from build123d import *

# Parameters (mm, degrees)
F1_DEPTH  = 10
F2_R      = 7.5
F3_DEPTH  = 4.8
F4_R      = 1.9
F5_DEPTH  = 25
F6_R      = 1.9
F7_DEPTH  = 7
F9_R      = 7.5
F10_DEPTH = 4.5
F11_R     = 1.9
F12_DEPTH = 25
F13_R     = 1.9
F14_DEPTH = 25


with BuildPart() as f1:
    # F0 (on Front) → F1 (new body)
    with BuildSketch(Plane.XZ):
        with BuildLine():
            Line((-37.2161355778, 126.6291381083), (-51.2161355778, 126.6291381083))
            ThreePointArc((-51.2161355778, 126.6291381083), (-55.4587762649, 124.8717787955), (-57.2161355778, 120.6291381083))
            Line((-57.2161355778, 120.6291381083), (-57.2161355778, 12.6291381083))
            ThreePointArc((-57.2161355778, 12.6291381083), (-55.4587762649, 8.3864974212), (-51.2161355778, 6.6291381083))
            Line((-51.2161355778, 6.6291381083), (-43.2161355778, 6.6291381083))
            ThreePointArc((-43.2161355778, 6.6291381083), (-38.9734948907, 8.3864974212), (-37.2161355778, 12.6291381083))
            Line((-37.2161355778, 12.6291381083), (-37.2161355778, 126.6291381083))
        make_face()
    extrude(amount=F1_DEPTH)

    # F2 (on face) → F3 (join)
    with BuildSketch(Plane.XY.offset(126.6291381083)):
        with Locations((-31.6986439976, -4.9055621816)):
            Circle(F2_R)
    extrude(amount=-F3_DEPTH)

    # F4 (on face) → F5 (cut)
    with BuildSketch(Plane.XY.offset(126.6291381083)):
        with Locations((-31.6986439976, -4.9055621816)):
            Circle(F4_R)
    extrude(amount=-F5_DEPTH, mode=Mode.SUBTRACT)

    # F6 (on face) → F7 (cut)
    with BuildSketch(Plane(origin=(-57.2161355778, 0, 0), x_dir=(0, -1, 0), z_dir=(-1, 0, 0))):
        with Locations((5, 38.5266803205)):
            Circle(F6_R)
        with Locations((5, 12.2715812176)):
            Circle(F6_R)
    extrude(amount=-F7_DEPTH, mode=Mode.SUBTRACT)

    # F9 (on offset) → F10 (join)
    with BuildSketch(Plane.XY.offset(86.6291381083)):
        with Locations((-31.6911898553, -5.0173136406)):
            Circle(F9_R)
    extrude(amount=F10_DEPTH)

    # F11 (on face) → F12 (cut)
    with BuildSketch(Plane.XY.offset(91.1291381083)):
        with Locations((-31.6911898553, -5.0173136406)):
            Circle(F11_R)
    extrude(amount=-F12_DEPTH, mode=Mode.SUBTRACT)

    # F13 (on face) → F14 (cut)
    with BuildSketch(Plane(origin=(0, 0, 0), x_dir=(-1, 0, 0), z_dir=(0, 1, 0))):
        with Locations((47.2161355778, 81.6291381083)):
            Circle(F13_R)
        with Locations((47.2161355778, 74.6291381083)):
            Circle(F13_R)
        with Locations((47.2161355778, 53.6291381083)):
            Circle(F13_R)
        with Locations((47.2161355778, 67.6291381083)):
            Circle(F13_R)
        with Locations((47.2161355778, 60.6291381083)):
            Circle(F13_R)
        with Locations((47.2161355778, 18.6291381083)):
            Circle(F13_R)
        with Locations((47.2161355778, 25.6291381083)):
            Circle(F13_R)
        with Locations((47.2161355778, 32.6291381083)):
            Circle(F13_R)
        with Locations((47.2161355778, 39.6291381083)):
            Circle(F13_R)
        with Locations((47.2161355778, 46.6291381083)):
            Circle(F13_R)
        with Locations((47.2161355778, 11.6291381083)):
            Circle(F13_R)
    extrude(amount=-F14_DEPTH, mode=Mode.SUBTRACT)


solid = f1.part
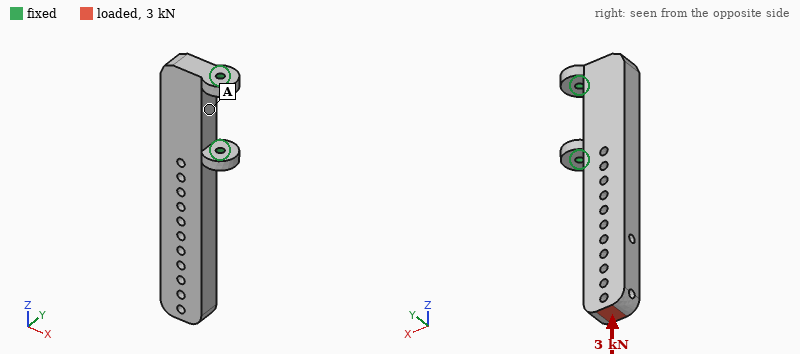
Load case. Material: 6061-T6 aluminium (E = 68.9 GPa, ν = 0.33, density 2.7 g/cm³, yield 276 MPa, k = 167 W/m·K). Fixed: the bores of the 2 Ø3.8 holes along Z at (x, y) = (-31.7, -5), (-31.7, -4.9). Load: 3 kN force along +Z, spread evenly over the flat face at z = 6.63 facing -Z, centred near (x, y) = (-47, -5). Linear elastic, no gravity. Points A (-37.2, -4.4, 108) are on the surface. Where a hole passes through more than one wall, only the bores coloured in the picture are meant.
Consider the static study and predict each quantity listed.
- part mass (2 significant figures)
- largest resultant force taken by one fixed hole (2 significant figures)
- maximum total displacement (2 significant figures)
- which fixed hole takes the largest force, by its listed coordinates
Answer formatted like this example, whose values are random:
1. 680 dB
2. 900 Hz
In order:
1. 64 g
2. 1.9 kN
3. 70 µm
4. (-31.7, -5)
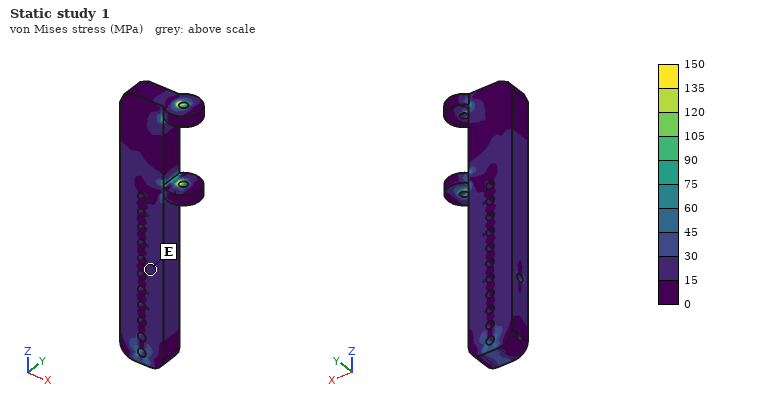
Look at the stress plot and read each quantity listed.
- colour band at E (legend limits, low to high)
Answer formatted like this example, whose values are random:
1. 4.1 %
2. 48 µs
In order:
1. 15 to 30 MPa
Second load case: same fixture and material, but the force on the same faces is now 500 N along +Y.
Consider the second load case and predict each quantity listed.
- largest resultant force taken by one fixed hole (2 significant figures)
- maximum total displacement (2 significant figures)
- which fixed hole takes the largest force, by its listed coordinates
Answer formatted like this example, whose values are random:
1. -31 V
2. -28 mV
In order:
1. 1.5 kN
2. 1.4 mm
3. (-31.7, -5)
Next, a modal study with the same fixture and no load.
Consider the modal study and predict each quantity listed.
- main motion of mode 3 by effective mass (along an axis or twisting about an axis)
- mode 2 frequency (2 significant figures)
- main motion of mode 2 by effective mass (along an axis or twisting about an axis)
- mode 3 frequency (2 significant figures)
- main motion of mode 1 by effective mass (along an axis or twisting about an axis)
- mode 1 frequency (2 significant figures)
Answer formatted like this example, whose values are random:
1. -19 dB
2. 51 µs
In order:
1. along Y
2. 1900 Hz
3. along X
4. 3500 Hz
5. along Y
6. 910 Hz
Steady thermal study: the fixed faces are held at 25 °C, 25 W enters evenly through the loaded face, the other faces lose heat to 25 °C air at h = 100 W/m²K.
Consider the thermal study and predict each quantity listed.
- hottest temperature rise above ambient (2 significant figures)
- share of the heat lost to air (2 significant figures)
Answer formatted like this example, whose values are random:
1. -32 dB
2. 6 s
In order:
1. 54 K
2. 64 %
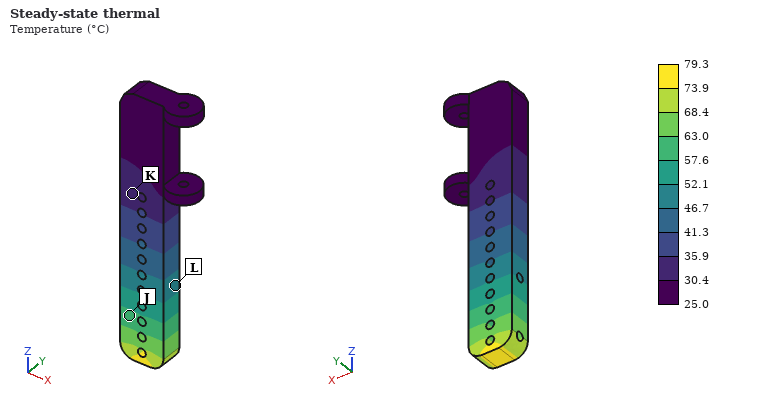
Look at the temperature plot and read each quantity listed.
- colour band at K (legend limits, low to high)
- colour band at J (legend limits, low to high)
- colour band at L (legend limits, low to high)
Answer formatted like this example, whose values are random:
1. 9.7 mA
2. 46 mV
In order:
1. 30.4 to 35.9 °C
2. 57.6 to 63.0 °C
3. 46.7 to 52.1 °C
